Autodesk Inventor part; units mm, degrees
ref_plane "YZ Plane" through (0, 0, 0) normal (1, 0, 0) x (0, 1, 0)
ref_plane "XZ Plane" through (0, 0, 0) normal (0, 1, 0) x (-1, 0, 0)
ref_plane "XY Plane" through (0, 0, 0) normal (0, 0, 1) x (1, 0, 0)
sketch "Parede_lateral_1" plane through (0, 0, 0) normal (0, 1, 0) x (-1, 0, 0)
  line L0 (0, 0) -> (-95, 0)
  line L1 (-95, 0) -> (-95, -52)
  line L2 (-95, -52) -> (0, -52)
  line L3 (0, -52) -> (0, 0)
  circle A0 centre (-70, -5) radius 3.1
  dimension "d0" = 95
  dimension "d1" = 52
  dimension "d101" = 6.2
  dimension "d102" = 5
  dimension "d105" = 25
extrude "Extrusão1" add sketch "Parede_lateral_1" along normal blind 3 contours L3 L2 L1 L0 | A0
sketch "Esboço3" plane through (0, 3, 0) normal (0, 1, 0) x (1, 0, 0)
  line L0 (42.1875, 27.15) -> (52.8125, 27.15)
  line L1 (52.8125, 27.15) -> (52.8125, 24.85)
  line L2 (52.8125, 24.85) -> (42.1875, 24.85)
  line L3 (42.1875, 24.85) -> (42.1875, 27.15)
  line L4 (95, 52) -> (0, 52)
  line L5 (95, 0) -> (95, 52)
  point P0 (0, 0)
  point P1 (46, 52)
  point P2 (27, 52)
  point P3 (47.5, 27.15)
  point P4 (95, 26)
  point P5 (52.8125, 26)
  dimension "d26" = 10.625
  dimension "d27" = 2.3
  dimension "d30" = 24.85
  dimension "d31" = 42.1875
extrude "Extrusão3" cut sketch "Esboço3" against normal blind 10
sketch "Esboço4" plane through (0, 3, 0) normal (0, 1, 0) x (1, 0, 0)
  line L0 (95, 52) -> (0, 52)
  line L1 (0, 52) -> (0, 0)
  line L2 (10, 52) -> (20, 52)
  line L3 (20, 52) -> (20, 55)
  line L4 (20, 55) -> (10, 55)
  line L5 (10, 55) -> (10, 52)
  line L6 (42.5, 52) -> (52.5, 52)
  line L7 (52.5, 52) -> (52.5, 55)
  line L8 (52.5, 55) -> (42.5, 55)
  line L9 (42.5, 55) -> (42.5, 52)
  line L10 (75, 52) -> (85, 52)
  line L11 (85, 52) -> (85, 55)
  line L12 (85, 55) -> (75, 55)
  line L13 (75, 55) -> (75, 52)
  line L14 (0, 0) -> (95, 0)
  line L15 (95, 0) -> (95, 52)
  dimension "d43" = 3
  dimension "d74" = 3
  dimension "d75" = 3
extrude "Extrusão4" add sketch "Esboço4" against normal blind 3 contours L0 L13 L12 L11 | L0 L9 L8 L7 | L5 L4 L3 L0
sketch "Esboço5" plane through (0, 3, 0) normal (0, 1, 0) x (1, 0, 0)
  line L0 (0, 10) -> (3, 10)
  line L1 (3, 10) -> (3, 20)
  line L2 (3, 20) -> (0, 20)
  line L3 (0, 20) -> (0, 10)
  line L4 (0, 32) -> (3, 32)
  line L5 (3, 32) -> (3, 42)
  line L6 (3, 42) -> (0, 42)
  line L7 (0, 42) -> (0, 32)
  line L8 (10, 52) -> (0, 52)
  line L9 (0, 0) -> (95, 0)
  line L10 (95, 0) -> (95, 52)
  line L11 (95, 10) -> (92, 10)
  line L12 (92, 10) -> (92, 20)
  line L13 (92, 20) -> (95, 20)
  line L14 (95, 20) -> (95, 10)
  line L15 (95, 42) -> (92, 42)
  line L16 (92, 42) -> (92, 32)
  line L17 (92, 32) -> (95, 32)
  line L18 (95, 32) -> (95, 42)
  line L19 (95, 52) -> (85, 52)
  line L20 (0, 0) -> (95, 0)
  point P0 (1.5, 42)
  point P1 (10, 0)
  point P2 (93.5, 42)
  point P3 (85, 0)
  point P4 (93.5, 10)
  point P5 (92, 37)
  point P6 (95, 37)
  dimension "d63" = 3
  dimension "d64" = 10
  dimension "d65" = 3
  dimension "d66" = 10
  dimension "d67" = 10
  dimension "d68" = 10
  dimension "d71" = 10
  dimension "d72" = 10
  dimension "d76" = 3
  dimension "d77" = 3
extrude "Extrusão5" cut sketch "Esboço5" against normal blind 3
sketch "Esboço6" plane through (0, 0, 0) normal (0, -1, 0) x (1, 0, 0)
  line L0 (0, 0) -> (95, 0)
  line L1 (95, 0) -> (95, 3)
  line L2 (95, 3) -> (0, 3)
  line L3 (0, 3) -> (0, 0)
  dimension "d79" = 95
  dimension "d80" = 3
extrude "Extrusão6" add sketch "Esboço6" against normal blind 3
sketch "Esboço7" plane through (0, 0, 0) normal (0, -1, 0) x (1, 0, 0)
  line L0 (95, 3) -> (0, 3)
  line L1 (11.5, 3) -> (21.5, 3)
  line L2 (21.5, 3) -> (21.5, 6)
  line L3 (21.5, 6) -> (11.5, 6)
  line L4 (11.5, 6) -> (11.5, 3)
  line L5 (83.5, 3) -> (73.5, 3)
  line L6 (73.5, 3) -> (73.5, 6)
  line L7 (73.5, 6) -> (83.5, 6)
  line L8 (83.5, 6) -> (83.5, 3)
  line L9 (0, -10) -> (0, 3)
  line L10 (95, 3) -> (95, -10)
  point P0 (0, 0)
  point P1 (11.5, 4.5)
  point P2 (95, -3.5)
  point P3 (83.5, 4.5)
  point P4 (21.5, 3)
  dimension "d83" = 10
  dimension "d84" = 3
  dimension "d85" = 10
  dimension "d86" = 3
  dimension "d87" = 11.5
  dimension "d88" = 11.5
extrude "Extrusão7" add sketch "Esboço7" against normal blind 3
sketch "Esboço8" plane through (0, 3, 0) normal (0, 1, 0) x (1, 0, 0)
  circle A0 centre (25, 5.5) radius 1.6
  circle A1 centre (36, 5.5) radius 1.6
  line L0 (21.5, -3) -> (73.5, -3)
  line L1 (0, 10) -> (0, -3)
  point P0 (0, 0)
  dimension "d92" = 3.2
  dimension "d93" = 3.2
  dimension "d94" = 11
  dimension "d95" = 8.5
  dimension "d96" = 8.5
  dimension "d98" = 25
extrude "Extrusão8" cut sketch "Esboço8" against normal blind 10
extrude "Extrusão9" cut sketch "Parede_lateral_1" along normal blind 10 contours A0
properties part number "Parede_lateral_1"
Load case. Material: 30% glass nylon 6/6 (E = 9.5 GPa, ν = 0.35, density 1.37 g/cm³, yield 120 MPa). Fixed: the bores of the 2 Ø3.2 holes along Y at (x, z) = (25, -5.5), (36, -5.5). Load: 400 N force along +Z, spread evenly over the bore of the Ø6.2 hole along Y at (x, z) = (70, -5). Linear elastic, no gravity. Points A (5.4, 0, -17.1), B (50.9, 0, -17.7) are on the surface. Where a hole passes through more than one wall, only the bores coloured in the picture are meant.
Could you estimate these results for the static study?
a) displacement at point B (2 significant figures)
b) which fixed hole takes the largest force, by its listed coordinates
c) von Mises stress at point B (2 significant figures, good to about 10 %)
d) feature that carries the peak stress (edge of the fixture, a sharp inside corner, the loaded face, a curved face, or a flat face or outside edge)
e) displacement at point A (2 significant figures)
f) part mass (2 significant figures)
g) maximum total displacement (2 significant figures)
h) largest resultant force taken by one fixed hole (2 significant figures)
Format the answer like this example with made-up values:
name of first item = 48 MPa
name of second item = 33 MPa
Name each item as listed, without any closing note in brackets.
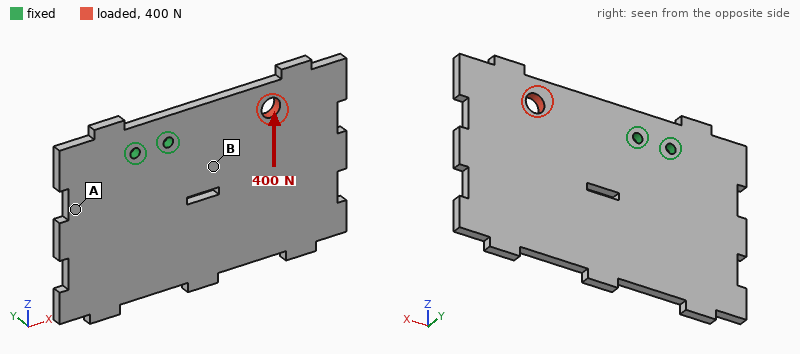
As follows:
displacement at point B = 0.15 mm
which fixed hole takes the largest force, by its listed coordinates = (36, -5.5)
von Mises stress at point B = 9.8 MPa
feature that carries the peak stress = edge of the fixture
displacement at point A = 0.15 mm
part mass = 21 g
maximum total displacement = 0.53 mm
largest resultant force taken by one fixed hole = 1.4 kN
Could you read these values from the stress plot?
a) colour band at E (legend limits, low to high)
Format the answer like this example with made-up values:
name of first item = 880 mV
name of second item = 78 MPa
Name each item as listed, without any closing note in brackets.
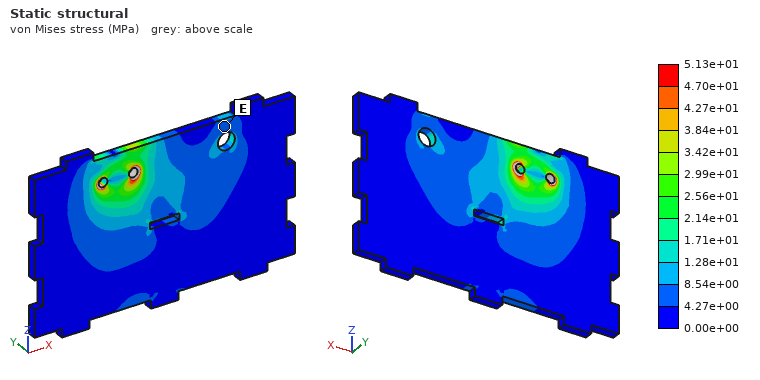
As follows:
colour band at E = 4.27e+00 to 8.54e+00 MPa
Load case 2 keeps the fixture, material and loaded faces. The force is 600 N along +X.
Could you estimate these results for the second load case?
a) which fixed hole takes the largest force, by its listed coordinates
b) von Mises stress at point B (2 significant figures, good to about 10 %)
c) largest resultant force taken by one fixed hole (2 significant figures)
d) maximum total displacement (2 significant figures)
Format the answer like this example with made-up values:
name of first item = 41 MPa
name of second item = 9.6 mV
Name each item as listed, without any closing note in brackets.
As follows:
which fixed hole takes the largest force, by its listed coordinates = (36, -5.5)
von Mises stress at point B = 4.5 MPa
largest resultant force taken by one fixed hole = 440 N
maximum total displacement = 69 µm
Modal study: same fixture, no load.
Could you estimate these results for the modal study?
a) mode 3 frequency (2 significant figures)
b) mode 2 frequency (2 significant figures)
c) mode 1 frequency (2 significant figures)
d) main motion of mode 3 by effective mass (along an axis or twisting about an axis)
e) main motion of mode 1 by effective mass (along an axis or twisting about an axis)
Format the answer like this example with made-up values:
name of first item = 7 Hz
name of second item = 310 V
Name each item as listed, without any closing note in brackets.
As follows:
mode 3 frequency = 830 Hz
mode 2 frequency = 470 Hz
mode 1 frequency = 270 Hz
main motion of mode 3 by effective mass = along Y
main motion of mode 1 by effective mass = along Y
